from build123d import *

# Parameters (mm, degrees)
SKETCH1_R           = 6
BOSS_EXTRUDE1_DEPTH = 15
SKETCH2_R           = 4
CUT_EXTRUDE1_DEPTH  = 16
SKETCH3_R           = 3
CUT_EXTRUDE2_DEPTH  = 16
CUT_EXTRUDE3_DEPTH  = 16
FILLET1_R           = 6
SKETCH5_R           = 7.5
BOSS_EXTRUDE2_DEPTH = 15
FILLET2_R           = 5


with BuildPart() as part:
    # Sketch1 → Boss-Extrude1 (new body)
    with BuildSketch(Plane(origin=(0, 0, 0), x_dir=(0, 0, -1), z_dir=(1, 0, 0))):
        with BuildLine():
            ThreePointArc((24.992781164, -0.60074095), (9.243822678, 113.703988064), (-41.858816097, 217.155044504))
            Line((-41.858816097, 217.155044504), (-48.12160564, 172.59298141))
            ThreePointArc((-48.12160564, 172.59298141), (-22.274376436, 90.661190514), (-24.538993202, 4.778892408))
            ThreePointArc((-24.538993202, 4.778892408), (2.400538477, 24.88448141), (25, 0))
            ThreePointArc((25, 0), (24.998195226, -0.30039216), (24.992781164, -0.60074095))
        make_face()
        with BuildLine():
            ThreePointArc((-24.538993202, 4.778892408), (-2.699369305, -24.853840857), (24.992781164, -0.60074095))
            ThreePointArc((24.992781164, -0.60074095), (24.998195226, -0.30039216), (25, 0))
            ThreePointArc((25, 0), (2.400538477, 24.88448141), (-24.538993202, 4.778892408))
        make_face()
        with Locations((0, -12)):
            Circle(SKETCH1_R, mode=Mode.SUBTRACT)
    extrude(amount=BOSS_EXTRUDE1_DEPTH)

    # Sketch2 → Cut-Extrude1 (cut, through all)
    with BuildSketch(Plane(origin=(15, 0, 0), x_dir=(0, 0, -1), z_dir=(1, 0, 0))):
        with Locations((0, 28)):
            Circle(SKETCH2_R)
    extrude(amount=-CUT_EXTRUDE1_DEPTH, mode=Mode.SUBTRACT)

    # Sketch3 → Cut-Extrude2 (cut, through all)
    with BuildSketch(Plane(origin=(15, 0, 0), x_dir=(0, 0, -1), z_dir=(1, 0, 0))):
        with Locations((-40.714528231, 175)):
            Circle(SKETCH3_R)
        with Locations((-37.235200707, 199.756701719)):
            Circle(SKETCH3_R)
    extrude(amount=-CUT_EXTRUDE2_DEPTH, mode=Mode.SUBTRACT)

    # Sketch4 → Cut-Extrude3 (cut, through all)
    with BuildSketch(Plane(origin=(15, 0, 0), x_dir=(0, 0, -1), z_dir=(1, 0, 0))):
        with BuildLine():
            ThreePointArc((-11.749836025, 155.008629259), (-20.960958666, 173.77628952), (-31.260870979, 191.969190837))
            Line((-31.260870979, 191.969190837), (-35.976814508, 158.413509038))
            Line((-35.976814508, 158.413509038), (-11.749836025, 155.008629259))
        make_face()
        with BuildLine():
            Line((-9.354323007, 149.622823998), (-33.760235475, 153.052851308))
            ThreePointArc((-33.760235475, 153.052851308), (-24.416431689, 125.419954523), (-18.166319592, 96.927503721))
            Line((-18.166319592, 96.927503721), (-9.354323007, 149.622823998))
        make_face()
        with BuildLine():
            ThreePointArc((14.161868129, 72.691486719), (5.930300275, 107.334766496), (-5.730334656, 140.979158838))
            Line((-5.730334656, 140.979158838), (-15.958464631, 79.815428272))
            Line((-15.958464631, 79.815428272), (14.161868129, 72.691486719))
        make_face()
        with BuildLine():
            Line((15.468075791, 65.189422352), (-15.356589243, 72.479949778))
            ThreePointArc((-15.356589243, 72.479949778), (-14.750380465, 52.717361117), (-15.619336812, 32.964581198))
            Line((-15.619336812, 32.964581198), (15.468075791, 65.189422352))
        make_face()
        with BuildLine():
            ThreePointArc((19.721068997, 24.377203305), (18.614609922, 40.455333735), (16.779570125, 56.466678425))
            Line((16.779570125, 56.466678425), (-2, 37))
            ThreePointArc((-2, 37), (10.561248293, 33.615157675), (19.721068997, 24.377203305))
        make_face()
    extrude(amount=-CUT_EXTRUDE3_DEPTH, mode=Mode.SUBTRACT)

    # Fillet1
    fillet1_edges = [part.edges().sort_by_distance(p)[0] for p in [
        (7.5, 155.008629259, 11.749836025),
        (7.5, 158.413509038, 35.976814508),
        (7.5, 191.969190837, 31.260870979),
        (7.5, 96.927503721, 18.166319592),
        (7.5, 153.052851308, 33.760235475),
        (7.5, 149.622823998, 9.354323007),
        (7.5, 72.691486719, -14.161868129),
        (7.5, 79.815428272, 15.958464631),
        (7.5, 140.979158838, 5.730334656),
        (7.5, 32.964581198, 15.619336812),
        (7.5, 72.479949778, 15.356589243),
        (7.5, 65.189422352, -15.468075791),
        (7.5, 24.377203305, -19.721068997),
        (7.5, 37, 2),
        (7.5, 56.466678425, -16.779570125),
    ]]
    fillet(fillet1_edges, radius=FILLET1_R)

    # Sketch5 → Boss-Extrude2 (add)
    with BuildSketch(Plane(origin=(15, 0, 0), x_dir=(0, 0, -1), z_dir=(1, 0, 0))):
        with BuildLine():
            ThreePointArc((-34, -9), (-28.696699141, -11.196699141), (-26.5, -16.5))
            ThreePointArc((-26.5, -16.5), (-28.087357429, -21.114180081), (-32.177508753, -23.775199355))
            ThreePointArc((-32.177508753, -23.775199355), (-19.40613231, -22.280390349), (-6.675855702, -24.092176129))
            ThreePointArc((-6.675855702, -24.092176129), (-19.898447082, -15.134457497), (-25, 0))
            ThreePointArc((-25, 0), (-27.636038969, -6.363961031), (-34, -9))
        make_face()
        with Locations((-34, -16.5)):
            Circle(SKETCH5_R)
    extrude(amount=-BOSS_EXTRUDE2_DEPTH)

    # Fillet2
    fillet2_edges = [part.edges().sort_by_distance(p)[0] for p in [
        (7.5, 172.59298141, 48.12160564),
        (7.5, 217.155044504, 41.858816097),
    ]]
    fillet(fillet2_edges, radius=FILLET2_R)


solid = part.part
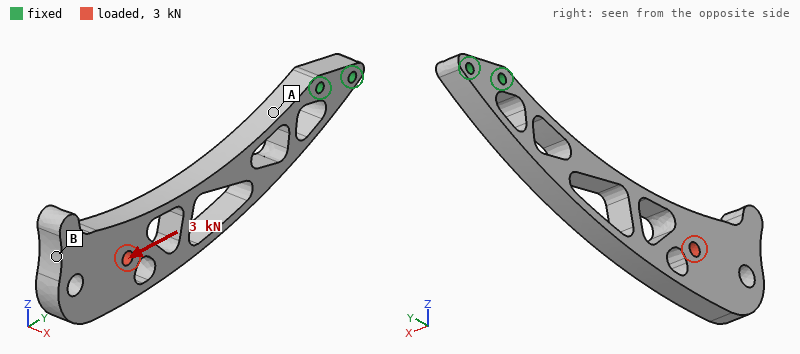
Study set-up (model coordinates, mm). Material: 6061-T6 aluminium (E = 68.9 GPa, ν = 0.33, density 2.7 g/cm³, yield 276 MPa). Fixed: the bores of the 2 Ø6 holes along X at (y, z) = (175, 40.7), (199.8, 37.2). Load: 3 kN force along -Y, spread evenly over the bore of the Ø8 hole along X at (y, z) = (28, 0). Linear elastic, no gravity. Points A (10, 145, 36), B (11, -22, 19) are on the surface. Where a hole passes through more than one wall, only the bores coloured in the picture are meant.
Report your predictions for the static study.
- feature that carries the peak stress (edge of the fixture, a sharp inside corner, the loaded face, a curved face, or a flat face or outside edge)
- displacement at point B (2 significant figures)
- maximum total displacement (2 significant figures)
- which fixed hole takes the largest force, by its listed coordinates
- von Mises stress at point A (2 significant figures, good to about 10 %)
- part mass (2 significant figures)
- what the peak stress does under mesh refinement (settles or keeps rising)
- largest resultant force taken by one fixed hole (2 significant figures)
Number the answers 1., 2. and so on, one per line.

1. edge of the fixture
2. 0.68 mm
3. 0.70 mm
4. (199.8, 37.2)
5. 18 MPa
6. 250 g
7. keeps rising
8. 4.7 kN
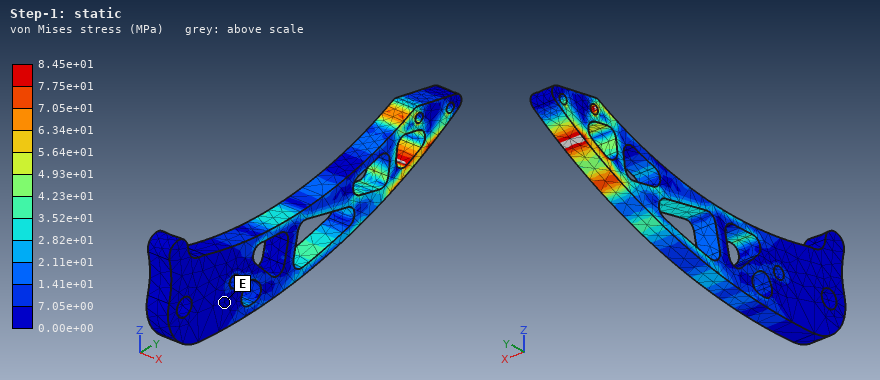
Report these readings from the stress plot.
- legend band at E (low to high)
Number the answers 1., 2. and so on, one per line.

1. 0.00e+00 to 7.05e+00 MPa
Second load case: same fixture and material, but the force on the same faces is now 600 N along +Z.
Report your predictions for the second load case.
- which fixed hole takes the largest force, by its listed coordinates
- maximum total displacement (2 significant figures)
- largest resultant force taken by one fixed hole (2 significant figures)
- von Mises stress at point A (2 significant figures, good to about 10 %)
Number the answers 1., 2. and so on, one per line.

1. (175, 40.7)
2. 0.74 mm
3. 3.7 kN
4. 40 MPa
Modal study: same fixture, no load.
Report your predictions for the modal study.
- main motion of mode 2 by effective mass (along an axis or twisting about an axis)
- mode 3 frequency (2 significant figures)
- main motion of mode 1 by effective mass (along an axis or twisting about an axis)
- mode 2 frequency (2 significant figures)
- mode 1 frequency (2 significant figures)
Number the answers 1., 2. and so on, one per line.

1. along Z
2. 780 Hz
3. along X
4. 380 Hz
5. 170 Hz
